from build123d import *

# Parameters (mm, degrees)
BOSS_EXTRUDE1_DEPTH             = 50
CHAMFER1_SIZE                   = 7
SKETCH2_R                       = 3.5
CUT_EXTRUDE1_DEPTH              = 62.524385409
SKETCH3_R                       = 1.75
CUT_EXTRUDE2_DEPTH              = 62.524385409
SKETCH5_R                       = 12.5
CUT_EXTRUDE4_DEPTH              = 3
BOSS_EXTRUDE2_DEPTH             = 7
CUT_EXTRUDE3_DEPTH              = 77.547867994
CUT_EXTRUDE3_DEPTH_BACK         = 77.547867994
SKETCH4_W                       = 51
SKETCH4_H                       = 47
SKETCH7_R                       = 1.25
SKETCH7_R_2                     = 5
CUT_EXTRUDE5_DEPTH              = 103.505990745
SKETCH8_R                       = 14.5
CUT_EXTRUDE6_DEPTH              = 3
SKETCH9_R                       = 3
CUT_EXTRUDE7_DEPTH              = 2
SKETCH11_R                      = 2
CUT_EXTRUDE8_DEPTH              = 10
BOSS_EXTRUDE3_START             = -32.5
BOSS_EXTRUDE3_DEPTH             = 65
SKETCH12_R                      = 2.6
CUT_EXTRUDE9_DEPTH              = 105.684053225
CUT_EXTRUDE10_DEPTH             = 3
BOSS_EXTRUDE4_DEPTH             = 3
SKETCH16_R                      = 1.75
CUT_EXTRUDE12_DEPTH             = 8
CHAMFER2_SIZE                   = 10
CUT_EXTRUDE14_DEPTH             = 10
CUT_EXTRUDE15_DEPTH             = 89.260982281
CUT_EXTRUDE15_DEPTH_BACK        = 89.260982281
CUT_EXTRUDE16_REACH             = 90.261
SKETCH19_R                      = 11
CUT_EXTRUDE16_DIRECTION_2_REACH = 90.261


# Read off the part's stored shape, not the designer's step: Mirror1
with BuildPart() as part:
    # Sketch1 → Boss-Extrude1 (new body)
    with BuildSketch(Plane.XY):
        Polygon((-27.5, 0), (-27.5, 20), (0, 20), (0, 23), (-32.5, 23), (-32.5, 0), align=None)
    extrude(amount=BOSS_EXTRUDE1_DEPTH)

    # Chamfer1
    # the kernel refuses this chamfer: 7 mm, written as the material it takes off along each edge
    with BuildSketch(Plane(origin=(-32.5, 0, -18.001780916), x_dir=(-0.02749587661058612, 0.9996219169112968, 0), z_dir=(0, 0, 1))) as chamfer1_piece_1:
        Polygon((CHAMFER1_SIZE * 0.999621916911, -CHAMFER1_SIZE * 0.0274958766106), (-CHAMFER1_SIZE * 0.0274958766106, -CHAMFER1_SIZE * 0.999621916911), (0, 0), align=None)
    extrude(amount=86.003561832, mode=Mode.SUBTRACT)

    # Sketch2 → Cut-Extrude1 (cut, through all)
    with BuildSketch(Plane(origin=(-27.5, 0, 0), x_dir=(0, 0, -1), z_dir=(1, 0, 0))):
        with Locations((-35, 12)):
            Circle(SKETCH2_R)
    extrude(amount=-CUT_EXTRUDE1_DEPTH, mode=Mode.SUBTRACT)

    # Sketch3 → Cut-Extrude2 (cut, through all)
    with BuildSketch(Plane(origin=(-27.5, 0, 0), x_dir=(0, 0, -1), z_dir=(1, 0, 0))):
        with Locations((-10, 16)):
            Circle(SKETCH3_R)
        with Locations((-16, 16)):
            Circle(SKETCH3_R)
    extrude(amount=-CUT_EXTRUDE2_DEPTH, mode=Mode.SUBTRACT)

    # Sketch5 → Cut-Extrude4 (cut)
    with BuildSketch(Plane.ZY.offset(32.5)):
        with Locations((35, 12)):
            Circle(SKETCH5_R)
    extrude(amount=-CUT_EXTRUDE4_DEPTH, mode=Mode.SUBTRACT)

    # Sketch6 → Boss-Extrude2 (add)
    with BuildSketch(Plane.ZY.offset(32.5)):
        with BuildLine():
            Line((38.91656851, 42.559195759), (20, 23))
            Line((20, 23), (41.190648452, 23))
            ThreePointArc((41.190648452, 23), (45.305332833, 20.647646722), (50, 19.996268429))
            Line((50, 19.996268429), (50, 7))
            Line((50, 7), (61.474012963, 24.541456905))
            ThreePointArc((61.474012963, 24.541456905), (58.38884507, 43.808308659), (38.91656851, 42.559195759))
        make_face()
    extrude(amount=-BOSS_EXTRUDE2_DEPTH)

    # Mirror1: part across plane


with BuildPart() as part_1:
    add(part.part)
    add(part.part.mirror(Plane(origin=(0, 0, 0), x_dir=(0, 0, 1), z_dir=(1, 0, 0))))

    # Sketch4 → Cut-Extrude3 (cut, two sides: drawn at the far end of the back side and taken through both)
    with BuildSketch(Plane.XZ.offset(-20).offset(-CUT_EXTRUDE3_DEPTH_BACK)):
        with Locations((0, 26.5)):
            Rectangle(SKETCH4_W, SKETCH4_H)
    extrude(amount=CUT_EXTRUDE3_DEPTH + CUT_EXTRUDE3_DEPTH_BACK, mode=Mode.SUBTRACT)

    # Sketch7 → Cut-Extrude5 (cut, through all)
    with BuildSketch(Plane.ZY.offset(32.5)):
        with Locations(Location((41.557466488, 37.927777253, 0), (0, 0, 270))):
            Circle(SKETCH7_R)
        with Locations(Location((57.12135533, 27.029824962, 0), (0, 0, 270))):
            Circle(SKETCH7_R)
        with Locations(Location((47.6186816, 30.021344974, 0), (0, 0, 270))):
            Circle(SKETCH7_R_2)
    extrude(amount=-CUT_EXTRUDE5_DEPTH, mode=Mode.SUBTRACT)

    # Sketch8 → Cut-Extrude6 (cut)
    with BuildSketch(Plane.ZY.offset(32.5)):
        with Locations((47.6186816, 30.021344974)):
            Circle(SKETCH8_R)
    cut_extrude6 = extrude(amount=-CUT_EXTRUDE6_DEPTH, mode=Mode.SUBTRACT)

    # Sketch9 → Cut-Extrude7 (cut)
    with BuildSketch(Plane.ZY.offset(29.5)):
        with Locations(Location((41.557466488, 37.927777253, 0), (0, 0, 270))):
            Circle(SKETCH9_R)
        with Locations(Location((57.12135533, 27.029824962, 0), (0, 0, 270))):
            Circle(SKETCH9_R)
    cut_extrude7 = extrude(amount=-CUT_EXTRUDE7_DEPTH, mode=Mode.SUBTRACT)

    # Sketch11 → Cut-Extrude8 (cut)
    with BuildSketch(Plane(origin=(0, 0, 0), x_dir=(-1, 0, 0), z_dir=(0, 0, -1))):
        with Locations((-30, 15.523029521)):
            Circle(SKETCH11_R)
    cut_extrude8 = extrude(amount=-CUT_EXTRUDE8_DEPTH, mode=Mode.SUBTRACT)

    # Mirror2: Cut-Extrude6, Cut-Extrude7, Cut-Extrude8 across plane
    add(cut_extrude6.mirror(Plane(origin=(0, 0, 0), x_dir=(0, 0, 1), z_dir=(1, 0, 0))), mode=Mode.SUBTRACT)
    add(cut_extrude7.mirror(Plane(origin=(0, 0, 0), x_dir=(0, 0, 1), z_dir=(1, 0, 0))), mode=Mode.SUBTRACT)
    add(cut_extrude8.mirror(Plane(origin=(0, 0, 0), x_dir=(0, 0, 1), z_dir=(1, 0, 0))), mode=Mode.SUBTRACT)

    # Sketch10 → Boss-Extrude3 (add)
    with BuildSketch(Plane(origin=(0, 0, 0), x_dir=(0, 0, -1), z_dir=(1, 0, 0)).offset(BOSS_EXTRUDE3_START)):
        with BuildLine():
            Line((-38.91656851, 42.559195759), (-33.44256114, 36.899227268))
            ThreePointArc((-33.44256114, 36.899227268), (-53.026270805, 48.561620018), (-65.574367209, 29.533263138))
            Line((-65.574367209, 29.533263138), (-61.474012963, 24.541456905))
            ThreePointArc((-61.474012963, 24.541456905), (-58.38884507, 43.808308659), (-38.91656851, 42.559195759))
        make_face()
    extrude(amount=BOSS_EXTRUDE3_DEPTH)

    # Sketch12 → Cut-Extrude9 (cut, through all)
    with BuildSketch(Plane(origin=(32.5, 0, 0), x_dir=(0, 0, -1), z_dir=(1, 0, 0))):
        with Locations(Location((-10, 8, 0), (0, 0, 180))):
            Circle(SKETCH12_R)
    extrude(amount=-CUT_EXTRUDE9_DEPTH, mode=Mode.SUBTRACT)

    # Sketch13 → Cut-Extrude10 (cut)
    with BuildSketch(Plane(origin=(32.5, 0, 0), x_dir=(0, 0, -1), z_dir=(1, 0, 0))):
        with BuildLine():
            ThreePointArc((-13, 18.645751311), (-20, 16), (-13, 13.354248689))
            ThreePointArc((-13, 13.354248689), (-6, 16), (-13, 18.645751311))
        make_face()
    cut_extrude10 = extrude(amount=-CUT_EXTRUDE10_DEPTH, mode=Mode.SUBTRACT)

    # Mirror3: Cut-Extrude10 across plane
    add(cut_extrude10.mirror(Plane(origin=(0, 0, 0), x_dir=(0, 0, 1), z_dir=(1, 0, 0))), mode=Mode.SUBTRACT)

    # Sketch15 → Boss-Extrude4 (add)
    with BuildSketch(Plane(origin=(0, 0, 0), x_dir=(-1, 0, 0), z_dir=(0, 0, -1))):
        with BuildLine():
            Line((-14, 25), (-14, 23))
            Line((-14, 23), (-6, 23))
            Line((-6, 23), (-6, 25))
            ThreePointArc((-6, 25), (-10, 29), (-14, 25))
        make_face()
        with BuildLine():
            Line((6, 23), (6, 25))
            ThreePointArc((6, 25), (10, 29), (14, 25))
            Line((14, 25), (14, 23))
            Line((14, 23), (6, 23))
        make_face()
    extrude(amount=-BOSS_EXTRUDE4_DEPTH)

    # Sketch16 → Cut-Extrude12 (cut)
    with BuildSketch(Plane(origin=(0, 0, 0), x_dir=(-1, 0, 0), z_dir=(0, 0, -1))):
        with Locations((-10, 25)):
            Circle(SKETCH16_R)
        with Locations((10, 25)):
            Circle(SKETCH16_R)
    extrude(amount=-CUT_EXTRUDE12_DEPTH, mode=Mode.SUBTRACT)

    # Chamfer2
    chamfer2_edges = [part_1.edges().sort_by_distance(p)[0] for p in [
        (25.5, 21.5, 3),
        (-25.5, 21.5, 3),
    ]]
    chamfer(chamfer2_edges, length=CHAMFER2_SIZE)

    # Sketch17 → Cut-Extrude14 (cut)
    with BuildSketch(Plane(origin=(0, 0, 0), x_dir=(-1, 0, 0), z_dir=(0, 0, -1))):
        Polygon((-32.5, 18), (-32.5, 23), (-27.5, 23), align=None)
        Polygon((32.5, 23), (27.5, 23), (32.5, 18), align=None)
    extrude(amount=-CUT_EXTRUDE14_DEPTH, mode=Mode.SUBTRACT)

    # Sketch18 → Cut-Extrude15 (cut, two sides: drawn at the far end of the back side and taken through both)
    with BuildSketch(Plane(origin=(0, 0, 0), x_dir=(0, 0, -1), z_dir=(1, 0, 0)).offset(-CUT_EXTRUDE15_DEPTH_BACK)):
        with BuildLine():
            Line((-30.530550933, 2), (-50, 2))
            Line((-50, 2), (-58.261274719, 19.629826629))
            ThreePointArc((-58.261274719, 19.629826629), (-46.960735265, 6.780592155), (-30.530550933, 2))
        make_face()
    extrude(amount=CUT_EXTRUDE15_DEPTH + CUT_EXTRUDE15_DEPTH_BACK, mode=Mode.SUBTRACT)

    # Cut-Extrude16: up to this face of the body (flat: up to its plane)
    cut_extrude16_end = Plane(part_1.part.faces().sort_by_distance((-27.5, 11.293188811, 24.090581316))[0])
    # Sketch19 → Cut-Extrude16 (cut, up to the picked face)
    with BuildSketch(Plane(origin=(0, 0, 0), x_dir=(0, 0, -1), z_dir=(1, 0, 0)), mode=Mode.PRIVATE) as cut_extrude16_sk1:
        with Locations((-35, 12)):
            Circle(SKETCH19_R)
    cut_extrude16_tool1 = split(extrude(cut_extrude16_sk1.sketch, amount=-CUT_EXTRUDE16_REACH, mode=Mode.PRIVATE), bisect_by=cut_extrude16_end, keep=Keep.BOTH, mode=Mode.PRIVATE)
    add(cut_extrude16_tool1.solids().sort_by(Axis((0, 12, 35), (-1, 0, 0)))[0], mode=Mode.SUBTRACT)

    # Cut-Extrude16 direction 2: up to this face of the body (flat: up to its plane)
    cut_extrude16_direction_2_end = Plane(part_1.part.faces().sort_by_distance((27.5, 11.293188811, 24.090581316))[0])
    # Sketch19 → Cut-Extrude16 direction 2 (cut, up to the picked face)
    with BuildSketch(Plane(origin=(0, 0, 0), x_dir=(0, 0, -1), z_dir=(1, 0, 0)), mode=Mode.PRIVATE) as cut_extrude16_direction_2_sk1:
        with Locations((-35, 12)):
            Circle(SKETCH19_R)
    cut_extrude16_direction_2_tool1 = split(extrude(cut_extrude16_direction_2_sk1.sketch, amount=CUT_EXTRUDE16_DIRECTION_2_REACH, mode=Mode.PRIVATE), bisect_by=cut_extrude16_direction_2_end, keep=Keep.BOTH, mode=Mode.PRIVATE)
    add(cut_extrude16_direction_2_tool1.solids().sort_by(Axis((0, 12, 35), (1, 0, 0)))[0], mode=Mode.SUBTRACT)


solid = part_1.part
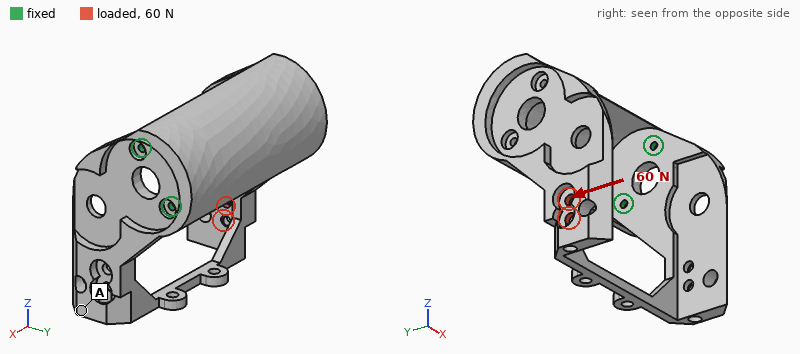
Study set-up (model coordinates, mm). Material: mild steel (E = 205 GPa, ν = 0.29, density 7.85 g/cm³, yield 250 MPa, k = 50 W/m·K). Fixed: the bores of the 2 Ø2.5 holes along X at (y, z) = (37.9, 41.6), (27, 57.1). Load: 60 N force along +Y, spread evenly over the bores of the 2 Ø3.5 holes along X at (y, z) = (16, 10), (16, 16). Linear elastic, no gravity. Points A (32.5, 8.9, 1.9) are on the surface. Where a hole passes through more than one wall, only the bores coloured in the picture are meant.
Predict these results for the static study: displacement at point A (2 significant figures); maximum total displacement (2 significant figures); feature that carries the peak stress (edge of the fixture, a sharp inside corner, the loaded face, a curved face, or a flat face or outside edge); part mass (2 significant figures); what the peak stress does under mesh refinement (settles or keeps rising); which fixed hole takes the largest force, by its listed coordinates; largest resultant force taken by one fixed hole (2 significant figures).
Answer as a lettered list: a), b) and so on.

a) 0.051 mm
b) 0.21 mm
c) edge of the fixture
d) 150 g
e) keeps rising
f) (37.9, 41.6)
g) 160 N
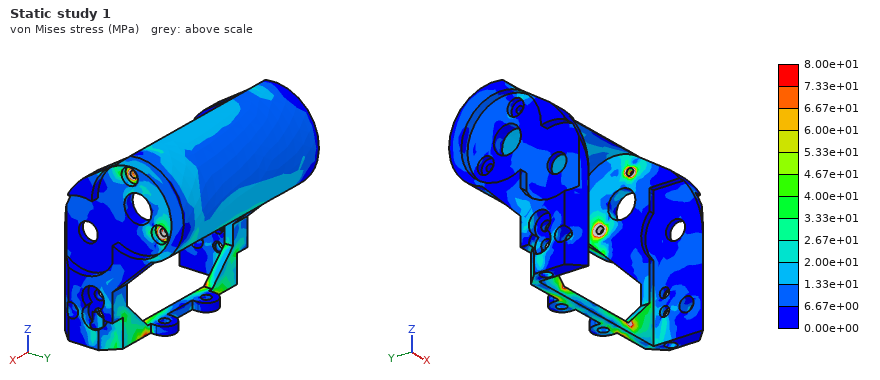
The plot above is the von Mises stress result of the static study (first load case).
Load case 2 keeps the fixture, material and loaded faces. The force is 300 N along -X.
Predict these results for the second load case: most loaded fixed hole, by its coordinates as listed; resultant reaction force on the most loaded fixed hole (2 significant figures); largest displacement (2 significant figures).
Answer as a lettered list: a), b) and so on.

a) (37.9, 41.6)
b) 460 N
c) 0.47 mm
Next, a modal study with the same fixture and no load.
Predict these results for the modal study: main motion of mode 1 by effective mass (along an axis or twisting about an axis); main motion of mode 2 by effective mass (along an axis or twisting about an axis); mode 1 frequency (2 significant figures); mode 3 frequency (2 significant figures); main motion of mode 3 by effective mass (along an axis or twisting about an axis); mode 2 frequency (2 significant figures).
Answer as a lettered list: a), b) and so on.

a) along Y
b) along Z
c) 450 Hz
d) 1600 Hz
e) along X
f) 520 Hz
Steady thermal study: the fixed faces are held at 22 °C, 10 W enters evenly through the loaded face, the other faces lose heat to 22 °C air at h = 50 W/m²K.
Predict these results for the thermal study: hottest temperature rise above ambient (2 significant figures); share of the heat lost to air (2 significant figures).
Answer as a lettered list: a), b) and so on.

a) 67 K
b) 95 %
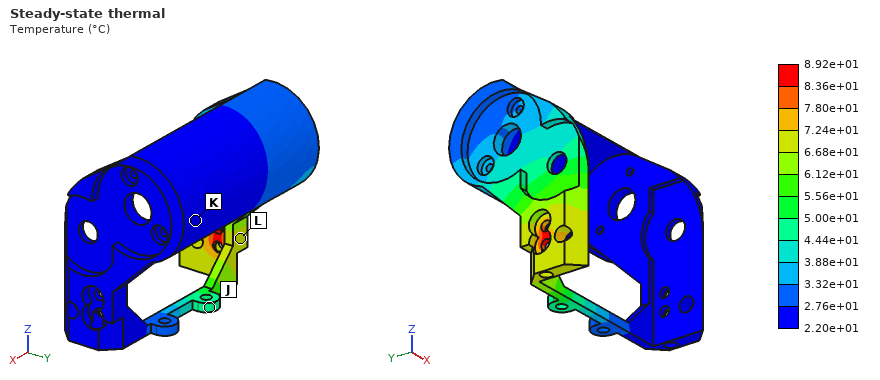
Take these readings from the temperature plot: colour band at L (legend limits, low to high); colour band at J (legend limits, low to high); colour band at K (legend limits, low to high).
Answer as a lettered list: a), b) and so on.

a) 6.68e+01 to 7.24e+01 °C
b) 4.44e+01 to 5.00e+01 °C
c) 2.20e+01 to 2.76e+01 °C
